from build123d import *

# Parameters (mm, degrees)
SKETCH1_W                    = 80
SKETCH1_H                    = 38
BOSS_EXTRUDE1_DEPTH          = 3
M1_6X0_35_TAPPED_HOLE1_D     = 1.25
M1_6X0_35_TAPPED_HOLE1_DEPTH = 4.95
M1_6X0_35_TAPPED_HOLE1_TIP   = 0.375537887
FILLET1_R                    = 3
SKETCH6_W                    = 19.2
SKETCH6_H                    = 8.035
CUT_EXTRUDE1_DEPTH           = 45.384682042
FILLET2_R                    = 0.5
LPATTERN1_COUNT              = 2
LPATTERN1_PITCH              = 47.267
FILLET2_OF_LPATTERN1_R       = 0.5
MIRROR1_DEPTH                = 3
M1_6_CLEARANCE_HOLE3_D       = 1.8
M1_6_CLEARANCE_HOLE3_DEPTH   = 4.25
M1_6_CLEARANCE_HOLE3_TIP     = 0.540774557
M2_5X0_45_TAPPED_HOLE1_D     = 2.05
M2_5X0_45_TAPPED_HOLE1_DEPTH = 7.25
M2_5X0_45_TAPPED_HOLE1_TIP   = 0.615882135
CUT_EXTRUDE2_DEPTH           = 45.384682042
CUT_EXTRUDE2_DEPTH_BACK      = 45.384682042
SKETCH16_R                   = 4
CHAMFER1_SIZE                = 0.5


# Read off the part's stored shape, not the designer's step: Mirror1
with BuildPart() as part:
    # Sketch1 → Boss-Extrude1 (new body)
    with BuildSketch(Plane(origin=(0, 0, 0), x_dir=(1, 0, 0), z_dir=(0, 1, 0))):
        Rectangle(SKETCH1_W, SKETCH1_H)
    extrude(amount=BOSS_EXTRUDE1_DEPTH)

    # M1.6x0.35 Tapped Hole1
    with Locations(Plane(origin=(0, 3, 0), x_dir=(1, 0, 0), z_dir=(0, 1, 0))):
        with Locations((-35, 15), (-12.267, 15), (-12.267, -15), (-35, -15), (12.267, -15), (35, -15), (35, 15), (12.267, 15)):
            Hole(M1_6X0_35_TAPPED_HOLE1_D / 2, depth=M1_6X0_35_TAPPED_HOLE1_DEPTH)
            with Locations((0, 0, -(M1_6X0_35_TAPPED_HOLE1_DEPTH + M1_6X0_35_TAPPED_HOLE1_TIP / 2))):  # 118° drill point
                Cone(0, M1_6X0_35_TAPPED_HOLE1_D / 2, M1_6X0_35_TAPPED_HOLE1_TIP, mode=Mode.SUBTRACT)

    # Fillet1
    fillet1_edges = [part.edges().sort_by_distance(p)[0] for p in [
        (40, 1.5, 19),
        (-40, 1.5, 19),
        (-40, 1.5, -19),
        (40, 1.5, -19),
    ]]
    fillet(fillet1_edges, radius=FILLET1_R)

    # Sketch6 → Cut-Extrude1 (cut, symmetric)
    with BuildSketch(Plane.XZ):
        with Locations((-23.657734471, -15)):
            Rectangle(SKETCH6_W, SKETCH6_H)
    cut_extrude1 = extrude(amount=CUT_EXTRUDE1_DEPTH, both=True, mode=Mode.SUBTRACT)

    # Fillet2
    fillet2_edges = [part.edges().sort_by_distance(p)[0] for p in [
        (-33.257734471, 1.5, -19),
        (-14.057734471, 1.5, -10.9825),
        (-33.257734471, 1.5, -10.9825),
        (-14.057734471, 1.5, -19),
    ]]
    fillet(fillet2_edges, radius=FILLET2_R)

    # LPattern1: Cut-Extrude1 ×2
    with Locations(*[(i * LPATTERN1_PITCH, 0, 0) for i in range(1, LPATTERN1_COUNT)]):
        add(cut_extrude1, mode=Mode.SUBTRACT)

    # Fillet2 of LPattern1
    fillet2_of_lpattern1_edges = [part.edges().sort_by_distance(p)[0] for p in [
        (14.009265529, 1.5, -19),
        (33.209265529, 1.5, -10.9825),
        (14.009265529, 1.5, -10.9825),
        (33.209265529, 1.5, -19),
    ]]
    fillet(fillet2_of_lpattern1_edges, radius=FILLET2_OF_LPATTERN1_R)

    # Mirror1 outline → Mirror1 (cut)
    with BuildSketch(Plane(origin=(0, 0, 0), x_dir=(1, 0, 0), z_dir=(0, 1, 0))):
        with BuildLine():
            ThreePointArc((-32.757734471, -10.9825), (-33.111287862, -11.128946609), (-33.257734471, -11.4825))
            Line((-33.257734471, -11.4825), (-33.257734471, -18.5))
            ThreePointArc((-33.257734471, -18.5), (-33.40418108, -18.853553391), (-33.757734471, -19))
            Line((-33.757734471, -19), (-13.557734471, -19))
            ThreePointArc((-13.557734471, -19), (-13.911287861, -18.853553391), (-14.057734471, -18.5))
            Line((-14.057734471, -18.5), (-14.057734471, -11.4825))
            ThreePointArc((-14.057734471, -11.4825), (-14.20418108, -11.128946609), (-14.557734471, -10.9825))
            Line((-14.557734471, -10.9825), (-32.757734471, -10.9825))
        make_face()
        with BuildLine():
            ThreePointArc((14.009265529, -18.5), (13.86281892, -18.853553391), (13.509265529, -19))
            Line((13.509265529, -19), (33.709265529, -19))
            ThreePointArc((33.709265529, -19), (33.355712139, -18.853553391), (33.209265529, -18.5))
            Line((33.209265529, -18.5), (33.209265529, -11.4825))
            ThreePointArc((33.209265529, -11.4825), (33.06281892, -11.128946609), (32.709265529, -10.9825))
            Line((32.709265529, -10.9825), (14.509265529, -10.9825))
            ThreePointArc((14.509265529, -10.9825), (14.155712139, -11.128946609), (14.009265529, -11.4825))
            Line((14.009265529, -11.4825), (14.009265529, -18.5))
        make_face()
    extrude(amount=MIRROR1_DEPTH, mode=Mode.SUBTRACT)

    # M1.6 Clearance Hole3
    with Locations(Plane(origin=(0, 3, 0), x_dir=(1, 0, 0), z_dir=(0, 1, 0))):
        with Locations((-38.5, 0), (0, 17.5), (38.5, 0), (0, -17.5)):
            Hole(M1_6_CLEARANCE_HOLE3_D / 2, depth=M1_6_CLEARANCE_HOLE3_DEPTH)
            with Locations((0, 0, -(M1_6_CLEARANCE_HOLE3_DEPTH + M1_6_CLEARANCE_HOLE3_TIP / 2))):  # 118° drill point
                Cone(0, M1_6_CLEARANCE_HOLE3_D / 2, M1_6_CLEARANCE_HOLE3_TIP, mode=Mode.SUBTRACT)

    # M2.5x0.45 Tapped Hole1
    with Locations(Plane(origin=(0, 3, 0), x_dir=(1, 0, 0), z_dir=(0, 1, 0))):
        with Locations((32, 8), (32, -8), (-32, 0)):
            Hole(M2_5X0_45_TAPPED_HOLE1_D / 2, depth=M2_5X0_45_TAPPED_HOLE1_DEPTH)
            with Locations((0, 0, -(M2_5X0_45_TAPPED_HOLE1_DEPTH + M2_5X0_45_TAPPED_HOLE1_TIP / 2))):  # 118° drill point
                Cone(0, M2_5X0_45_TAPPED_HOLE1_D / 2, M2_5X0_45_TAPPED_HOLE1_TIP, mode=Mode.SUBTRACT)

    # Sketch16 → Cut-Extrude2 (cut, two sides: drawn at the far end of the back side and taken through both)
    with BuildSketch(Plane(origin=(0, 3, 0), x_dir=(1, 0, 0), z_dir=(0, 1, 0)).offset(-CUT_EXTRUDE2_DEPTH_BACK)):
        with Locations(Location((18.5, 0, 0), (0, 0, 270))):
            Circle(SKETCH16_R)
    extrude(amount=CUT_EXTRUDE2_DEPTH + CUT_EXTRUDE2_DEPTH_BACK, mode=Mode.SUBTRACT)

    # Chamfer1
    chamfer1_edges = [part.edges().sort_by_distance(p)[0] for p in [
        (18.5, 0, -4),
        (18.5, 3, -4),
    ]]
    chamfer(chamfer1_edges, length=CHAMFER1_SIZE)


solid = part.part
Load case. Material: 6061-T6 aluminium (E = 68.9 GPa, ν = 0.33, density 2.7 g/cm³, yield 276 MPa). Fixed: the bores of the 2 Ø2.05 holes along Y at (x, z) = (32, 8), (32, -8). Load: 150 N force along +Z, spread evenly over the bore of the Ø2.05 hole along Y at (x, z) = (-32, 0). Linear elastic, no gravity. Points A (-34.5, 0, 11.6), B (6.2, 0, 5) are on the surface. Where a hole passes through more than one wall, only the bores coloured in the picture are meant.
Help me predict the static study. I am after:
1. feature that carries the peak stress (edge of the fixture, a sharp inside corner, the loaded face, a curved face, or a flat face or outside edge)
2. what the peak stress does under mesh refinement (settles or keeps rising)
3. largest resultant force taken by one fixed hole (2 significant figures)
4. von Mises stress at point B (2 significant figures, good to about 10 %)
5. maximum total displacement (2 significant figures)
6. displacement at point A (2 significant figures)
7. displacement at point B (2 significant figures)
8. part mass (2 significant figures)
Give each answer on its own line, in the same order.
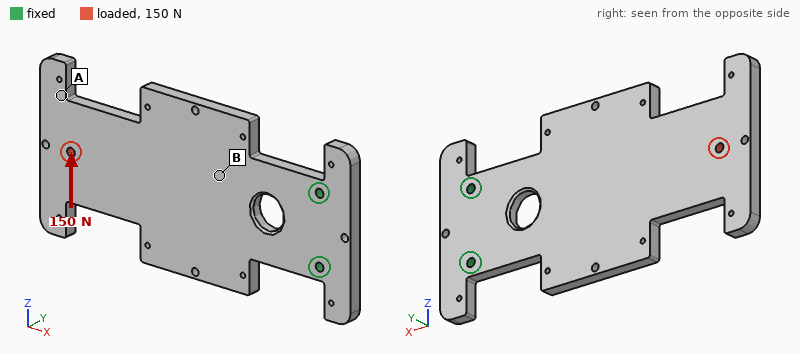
edge of the fixture
keeps rising
580 N
11 MPa
86 µm
77 µm
22 µm
19 g
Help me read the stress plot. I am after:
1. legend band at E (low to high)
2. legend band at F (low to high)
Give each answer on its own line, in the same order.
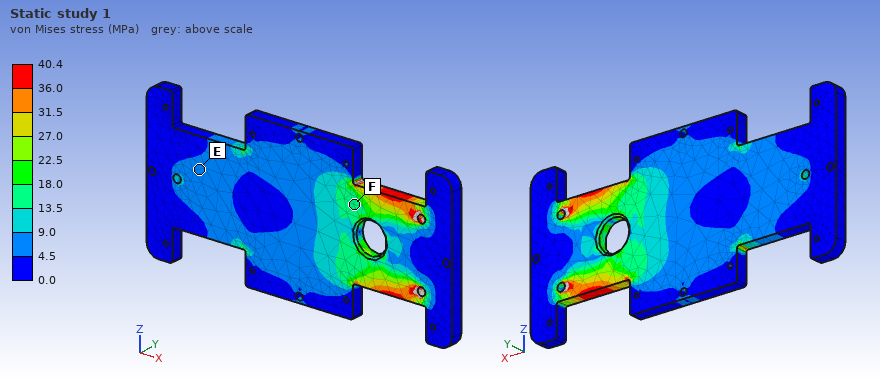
4.5 to 9.0 MPa
13.5 to 18.0 MPa
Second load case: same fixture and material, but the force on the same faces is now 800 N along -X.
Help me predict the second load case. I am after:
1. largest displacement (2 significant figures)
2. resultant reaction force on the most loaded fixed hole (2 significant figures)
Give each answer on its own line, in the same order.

14 µm
400 N
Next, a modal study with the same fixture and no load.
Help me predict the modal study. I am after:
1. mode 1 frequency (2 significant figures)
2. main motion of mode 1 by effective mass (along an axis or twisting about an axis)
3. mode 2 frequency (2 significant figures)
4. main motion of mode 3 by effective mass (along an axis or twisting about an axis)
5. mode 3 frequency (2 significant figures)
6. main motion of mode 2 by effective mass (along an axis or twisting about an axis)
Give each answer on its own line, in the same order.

390 Hz
along Y
1800 Hz
along Y
2500 Hz
twisting about X
